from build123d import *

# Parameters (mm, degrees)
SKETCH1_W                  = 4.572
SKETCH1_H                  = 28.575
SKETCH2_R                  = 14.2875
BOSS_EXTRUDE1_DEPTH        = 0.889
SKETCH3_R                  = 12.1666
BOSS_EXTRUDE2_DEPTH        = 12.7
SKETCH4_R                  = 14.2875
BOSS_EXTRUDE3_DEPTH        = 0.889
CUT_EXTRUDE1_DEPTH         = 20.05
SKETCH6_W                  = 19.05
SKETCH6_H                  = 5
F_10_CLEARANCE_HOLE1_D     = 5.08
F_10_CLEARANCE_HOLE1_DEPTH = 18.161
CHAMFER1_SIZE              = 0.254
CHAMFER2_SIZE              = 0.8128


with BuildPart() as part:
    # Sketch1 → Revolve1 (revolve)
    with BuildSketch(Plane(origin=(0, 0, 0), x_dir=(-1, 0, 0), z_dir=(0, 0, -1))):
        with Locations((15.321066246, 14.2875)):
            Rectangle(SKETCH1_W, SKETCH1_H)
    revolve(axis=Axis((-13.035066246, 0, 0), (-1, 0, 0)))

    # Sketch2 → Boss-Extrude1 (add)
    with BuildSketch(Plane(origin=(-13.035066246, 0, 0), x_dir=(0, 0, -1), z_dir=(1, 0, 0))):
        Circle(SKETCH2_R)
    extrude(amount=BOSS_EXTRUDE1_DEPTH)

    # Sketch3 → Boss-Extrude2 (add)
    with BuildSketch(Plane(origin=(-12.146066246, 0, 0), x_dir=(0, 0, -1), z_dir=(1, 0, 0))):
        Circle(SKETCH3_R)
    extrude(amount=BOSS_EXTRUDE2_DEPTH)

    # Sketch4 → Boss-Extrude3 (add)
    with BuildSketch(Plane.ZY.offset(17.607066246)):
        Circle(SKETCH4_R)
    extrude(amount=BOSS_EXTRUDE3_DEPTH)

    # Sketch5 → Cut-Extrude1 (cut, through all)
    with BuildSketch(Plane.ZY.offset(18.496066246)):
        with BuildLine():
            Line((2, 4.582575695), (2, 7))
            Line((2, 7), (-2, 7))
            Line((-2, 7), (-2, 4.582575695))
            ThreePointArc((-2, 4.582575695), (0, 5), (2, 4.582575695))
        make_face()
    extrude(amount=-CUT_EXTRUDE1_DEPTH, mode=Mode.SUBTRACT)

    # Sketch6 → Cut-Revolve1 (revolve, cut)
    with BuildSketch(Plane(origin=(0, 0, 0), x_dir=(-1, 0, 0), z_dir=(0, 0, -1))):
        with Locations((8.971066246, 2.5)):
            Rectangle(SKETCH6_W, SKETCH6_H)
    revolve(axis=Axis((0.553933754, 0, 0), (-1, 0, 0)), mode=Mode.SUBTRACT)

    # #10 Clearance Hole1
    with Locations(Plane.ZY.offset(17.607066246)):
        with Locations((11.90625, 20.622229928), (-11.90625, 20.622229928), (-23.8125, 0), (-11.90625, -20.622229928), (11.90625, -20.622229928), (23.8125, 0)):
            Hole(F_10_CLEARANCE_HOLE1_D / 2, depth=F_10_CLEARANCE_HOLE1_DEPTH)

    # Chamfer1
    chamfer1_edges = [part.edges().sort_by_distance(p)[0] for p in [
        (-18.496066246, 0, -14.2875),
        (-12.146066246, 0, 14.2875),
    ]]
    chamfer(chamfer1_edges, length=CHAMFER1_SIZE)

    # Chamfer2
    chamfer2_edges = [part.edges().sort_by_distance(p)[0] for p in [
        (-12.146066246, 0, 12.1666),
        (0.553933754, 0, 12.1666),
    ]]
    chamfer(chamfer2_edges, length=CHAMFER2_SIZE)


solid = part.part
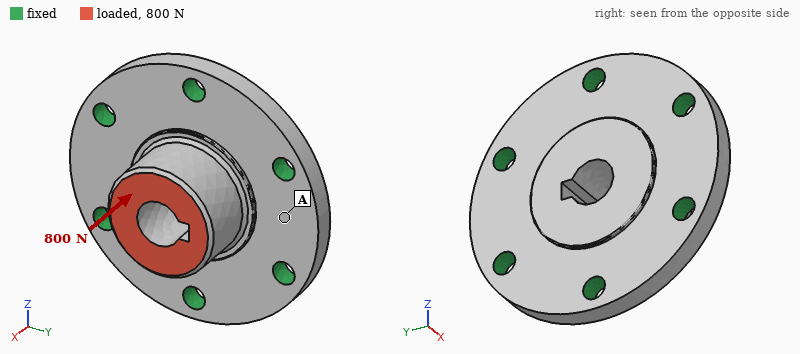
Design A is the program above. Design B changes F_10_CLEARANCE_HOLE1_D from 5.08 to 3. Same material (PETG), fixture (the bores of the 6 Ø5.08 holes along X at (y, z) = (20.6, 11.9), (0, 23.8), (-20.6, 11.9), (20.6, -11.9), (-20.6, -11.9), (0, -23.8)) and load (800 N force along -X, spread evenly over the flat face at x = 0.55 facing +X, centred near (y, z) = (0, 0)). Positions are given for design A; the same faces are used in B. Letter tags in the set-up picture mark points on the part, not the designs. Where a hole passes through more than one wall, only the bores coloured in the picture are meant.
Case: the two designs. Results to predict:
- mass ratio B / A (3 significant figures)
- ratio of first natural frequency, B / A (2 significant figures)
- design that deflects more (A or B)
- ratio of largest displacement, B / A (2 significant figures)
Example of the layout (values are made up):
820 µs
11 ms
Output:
1.02
0.86
B
1.3
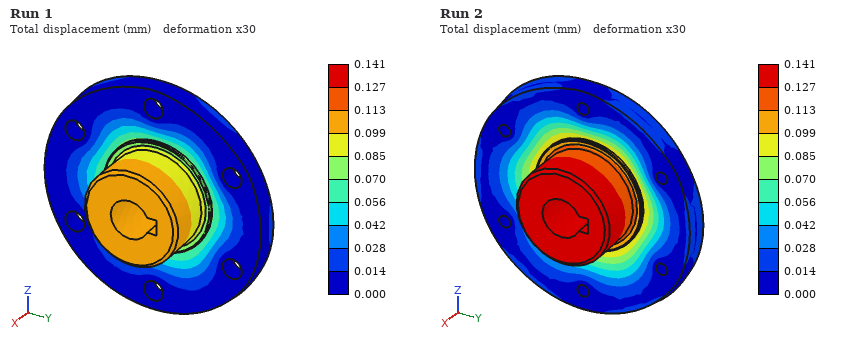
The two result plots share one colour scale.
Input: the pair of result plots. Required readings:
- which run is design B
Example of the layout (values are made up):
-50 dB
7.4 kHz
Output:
Run 2
